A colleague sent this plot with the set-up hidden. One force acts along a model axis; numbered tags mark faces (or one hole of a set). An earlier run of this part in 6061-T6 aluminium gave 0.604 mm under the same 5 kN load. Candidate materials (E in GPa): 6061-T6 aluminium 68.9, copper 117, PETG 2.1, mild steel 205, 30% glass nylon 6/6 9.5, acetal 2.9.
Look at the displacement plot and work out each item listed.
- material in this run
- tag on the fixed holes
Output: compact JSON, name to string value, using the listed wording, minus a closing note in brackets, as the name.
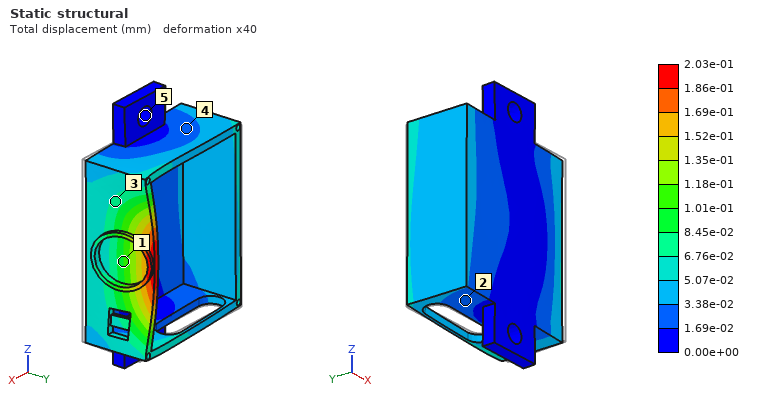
{"material in this run": "mild steel", "tag on the fixed holes": "5"}
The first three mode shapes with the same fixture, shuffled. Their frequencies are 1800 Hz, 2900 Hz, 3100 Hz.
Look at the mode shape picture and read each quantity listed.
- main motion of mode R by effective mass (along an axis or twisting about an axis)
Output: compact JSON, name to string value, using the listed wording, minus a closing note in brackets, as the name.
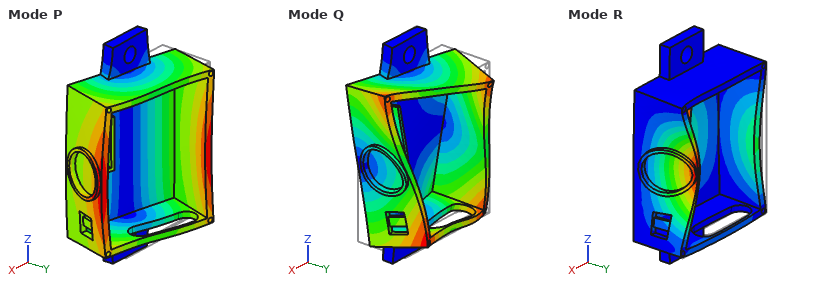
{"main motion of mode R by effective mass": "along Y"}
